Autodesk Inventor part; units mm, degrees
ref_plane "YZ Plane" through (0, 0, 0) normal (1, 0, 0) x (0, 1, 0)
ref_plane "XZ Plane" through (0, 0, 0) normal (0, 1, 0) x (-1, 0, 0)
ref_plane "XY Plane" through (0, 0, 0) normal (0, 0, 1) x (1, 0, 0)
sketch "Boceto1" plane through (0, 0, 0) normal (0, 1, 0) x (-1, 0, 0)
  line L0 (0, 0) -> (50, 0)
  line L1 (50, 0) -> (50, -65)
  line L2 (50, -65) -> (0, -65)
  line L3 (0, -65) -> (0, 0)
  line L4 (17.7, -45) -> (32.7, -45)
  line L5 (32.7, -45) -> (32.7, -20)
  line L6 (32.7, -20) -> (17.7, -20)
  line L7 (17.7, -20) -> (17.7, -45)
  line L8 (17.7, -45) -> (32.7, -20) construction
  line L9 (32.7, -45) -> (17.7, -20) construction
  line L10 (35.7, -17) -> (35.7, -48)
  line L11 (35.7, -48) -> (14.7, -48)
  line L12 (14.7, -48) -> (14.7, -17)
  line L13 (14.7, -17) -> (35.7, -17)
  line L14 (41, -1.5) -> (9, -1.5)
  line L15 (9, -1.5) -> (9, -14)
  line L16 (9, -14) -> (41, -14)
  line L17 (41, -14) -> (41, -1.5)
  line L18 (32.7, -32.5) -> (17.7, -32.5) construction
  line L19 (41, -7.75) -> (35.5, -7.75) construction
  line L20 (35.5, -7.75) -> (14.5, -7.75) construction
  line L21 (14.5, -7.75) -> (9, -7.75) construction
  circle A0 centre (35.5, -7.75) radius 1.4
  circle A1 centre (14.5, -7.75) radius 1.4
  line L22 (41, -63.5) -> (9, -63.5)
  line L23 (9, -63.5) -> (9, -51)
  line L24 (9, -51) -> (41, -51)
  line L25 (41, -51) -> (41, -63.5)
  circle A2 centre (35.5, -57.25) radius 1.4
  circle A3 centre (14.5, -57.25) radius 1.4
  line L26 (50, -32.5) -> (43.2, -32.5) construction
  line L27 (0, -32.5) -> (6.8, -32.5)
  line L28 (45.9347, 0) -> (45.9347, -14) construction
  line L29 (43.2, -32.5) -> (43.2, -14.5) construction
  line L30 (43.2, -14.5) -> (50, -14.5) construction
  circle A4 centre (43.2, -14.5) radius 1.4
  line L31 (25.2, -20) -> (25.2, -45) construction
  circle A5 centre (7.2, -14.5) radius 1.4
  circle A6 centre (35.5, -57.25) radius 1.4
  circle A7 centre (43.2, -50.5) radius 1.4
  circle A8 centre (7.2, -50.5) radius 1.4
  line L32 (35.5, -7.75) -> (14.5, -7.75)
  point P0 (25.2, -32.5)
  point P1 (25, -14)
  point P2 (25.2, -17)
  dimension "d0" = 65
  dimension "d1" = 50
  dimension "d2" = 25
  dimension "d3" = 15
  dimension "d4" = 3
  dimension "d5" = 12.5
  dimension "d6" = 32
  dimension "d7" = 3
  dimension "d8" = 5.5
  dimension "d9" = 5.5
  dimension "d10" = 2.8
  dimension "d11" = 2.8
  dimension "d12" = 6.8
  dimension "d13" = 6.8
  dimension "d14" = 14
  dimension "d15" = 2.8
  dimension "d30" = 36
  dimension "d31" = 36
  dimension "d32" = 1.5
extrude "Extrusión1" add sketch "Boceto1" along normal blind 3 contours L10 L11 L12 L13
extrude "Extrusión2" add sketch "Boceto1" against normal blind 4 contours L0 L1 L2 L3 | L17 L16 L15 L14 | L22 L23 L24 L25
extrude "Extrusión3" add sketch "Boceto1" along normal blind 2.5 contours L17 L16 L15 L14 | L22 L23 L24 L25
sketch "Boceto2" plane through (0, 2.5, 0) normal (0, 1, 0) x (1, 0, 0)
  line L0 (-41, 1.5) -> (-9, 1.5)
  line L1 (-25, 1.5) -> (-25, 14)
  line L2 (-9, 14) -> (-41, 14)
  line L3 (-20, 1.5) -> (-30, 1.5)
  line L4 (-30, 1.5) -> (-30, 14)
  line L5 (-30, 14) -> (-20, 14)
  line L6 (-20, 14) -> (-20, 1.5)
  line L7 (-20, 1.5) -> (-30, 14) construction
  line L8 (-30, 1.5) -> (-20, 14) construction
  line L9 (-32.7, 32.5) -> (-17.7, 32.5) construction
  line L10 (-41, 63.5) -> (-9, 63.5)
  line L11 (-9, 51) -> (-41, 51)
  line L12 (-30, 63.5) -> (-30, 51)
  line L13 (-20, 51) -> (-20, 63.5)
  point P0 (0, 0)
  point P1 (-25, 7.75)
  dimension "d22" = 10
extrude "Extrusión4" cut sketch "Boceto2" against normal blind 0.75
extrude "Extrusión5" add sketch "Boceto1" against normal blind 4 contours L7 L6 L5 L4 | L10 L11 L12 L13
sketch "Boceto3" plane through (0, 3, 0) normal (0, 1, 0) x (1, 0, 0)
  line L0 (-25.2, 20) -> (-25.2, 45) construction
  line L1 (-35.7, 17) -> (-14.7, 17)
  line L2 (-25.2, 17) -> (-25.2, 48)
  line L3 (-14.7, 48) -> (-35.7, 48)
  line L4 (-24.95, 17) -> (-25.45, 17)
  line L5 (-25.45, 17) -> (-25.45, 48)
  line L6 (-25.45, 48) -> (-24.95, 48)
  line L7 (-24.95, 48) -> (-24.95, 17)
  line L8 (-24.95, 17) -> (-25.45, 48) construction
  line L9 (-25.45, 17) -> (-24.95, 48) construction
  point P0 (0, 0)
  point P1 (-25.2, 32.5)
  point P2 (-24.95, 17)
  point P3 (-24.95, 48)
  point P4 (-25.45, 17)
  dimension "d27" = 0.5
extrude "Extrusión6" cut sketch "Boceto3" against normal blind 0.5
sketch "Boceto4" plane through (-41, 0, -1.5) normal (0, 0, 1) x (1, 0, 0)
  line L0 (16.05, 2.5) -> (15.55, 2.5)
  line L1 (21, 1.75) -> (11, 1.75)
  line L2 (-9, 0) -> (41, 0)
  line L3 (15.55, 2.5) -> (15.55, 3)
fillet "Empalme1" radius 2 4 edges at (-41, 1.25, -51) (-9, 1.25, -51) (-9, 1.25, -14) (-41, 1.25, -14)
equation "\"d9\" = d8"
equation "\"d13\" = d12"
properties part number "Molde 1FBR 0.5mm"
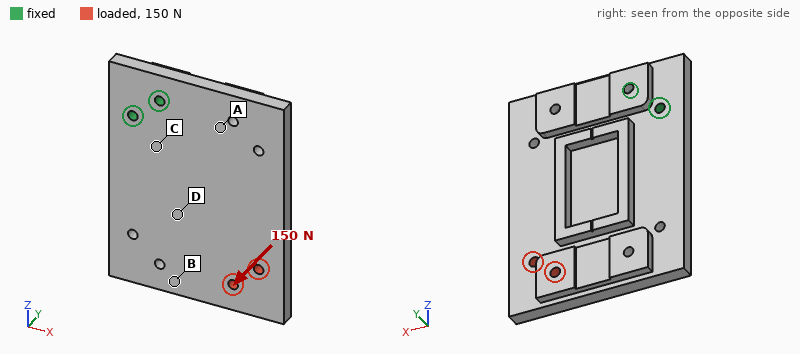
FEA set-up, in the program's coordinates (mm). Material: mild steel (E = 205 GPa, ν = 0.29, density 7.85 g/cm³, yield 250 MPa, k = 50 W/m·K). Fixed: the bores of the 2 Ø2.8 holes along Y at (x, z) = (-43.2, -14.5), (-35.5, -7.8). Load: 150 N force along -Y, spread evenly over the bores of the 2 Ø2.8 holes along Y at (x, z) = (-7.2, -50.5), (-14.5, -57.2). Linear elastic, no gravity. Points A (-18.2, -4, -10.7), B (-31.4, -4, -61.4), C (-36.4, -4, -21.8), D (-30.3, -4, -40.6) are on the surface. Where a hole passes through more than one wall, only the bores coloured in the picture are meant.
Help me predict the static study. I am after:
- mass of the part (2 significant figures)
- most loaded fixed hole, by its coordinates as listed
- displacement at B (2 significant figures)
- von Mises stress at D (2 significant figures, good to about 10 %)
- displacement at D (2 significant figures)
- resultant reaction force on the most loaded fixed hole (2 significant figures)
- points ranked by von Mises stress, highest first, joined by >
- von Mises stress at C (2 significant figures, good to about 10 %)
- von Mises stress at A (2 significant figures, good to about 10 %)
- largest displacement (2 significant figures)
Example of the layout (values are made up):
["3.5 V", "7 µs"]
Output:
["120 g", "(-43.2, -14.5)", "0.096 mm", "15 MPa", "0.050 mm", "140 N", "C > A > D > B", "39 MPa", "27 MPa", "0.16 mm"]
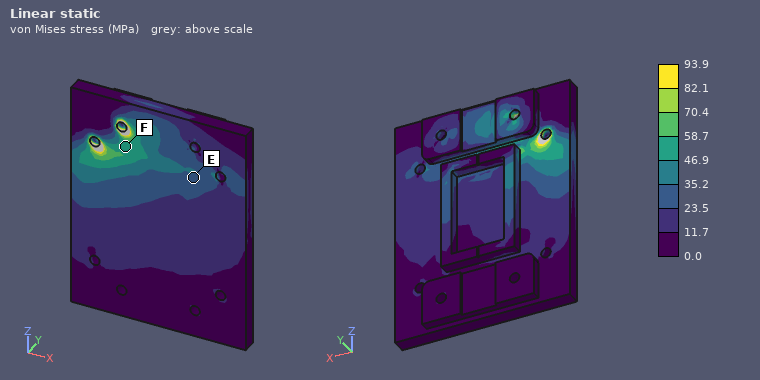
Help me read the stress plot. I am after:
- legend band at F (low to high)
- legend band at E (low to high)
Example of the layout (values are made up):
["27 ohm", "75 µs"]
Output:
["46.9 to 58.7 MPa", "23.5 to 35.2 MPa"]
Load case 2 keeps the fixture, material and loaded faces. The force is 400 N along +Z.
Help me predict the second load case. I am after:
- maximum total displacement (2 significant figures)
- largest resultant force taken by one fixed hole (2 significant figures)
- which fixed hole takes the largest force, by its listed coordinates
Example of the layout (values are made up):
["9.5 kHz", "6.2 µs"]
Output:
["12 µm", "1.1 kN", "(-35.5, -7.8)"]
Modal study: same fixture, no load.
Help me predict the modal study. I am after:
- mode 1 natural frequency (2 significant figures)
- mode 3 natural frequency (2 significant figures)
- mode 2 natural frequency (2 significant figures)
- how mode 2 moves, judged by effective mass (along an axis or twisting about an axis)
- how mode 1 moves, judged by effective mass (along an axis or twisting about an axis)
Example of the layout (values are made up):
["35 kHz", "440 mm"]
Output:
["950 Hz", "3300 Hz", "2400 Hz", "twisting about Z", "along Y"]
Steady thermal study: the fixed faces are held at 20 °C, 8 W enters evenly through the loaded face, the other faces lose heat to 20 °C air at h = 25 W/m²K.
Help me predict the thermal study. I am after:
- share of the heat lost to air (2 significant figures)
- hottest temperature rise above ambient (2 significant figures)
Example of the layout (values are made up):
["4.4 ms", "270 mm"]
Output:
["41 %", "37 K"]
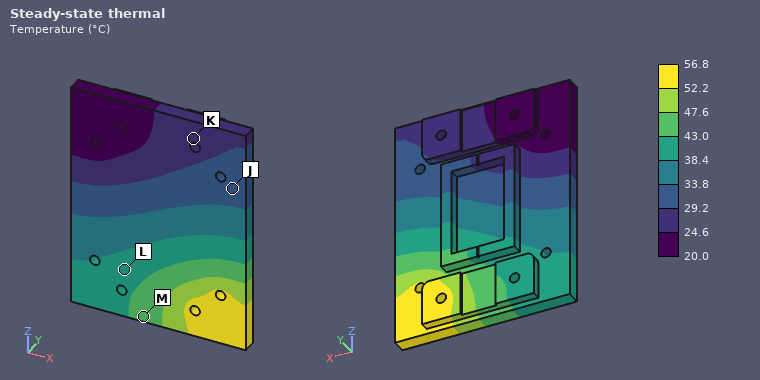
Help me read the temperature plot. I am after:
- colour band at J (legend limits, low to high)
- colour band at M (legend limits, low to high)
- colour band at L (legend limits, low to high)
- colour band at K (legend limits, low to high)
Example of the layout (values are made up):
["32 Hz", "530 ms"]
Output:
["29.2 to 33.8 °C", "43.0 to 47.6 °C", "38.4 to 43.0 °C", "24.6 to 29.2 °C"]
